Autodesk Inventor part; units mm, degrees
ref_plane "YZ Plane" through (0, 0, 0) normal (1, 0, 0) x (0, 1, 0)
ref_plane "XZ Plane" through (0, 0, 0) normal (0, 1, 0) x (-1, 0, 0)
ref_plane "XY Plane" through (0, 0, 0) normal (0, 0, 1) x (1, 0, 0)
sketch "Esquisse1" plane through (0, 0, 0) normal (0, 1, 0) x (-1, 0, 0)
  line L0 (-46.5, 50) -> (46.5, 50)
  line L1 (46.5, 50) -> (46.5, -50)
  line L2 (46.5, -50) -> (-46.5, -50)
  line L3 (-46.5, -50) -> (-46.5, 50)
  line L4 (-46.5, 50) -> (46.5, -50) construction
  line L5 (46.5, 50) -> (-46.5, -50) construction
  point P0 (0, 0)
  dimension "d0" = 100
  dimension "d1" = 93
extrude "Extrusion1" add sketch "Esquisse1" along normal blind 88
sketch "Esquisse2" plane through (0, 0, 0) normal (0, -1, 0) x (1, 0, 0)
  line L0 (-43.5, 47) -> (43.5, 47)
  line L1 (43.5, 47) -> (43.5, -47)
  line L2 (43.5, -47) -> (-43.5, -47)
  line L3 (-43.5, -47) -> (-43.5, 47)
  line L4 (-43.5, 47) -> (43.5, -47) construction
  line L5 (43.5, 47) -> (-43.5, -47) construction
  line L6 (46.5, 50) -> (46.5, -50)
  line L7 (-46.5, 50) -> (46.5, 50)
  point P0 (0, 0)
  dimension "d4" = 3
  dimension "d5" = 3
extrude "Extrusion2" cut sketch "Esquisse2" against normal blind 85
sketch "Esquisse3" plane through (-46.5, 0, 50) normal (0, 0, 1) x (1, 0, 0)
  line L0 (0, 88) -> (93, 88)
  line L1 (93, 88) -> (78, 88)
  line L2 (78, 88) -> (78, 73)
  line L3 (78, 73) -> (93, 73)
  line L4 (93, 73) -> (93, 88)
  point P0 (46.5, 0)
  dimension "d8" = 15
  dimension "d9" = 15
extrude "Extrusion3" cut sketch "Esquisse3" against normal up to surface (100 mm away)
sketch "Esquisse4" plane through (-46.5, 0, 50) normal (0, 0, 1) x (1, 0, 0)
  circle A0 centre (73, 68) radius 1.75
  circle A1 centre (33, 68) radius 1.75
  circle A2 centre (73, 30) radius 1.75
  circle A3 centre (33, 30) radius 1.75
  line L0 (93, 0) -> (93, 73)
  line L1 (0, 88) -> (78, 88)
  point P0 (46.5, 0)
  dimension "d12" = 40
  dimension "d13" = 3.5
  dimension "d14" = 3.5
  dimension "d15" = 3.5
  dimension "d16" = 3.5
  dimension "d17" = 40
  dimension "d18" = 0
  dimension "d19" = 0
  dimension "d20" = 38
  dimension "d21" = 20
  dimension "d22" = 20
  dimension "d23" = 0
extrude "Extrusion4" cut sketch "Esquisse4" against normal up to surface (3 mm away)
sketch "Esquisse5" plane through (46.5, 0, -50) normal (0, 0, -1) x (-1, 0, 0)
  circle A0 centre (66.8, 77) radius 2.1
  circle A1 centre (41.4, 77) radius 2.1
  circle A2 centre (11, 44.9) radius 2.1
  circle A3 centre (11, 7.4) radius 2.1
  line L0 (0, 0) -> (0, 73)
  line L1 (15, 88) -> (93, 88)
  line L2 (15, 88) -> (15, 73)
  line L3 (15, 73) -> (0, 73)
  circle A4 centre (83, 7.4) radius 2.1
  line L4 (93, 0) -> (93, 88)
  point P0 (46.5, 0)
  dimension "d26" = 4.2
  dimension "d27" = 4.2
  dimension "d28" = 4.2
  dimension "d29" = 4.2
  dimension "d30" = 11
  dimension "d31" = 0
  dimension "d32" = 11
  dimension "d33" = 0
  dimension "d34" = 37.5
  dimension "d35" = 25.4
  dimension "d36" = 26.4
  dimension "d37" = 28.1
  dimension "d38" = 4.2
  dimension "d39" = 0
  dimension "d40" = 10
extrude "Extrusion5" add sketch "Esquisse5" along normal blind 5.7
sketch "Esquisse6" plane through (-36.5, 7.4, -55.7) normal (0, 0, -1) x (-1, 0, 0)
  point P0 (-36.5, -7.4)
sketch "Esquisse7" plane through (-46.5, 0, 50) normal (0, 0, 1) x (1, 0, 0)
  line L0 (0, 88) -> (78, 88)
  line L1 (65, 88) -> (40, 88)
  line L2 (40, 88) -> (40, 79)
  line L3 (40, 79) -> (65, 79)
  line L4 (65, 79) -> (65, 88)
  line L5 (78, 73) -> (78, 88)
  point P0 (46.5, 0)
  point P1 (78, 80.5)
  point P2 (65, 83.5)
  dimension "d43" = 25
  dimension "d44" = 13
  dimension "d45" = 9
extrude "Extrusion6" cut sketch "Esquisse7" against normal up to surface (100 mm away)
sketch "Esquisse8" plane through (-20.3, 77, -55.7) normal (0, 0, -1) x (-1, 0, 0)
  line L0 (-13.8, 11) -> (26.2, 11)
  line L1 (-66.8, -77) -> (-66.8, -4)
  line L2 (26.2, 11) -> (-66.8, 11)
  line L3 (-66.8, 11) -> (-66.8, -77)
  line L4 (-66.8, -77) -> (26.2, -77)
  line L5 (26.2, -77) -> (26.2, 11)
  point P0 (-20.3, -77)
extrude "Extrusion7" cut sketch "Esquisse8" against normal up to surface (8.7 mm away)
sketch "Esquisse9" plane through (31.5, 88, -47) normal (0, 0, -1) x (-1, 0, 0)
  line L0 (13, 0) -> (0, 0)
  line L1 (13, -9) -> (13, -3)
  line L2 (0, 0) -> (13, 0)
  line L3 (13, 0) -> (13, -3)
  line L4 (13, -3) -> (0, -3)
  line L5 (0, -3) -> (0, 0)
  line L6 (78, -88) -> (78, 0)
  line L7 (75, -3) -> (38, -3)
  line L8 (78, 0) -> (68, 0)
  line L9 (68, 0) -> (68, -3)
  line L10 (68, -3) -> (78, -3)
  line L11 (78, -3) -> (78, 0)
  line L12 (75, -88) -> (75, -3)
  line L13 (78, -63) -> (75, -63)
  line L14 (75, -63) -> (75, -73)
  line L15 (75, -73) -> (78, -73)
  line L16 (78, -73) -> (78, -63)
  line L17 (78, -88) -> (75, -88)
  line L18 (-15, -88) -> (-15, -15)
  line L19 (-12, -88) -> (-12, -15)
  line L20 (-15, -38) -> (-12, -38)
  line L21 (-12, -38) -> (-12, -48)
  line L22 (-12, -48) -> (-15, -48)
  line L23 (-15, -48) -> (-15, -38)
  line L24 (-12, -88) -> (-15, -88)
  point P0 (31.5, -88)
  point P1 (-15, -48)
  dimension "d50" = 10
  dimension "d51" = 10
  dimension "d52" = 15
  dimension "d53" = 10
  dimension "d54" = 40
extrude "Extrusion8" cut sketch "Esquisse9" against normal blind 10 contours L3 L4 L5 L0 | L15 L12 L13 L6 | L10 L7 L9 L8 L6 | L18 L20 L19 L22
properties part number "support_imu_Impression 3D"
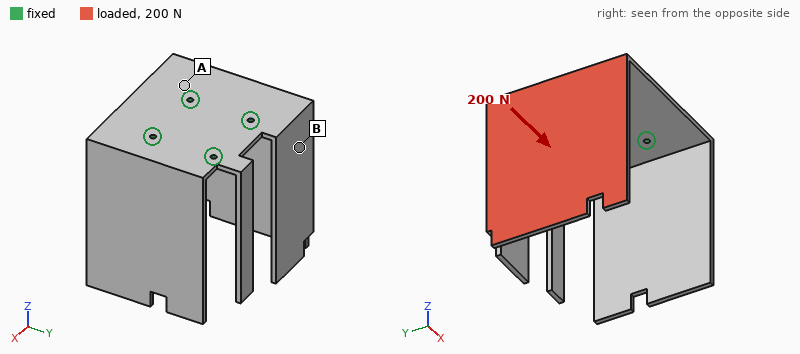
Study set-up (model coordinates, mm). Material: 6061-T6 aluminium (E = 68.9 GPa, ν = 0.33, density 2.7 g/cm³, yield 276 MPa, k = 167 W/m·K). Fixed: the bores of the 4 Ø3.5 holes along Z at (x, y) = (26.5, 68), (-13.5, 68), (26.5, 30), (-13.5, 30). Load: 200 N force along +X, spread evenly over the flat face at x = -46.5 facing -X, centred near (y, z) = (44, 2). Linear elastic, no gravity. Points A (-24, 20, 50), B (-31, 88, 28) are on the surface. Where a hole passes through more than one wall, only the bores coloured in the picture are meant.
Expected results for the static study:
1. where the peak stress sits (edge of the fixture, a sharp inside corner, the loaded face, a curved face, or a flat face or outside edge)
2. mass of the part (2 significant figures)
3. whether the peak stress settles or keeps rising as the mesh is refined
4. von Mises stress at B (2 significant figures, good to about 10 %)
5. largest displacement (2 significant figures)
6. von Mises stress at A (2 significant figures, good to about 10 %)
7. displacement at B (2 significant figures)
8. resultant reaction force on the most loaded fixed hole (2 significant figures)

edge of the fixture
220 g
keeps rising
13 MPa
1.8 mm
38 MPa
0.30 mm
90 N
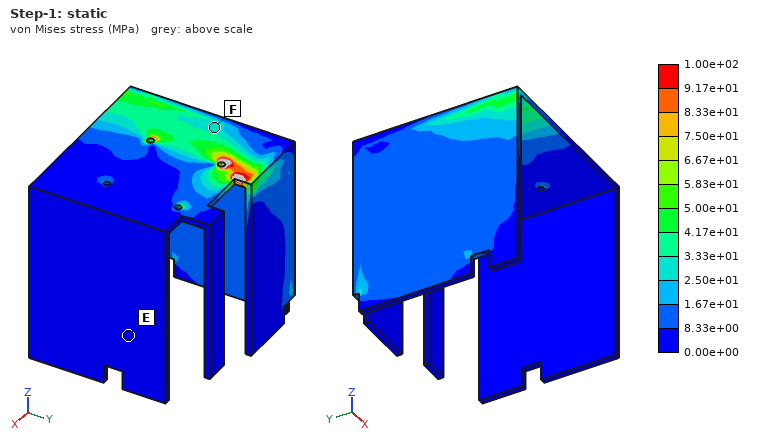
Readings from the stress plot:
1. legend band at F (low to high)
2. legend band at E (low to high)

2.50e+01 to 3.33e+01 MPa
0.00e+00 to 8.33e+00 MPa
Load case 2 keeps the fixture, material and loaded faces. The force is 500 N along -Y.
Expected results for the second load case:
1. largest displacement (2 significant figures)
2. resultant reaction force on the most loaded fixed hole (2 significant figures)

1.6 mm
650 N
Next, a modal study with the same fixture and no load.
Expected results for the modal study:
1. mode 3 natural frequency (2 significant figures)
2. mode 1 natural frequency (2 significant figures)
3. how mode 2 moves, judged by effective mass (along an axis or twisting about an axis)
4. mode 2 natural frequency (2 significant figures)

260 Hz
210 Hz
along X
230 Hz
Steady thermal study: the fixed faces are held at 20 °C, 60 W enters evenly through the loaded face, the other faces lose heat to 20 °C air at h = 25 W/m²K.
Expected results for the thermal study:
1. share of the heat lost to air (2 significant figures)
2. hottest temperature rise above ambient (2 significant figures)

37 %
66 K
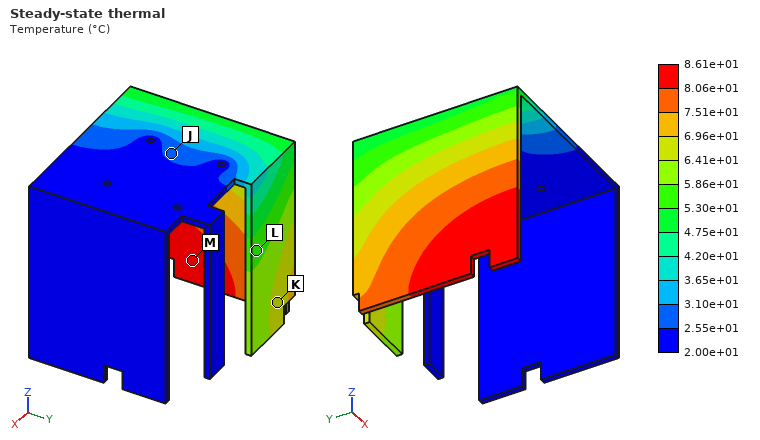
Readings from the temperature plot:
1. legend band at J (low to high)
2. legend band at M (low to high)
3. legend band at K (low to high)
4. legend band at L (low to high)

2.55e+01 to 3.10e+01 °C
8.06e+01 to 8.61e+01 °C
6.41e+01 to 6.96e+01 °C
5.30e+01 to 5.86e+01 °C
